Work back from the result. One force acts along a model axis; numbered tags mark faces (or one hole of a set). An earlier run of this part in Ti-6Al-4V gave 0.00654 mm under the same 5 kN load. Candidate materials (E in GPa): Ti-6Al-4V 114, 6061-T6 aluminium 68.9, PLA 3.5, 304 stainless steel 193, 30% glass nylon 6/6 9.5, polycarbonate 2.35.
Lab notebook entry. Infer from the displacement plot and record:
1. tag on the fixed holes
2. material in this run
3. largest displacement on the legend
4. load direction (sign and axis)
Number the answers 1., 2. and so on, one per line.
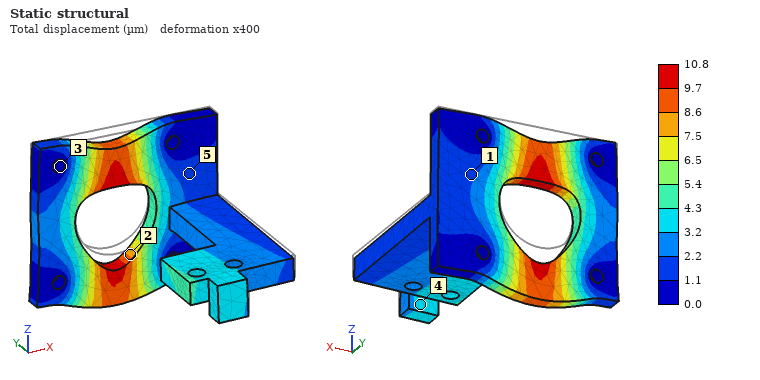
1. 3
2. 6061-T6 aluminium
3. 10.8 µm
4. -Z
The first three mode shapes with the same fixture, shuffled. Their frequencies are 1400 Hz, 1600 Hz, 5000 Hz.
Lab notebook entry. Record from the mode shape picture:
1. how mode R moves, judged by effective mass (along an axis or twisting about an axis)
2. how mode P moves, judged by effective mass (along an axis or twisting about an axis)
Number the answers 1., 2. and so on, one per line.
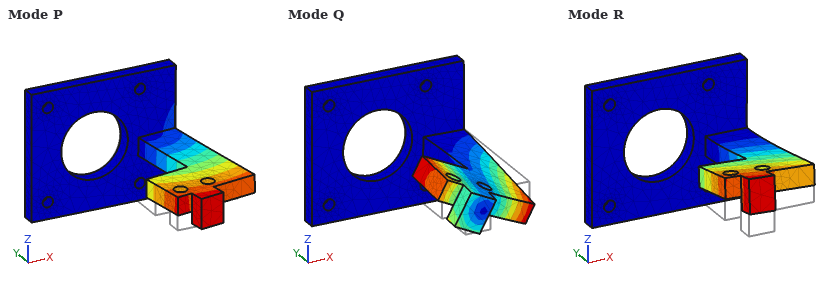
1. along Z
2. along X
